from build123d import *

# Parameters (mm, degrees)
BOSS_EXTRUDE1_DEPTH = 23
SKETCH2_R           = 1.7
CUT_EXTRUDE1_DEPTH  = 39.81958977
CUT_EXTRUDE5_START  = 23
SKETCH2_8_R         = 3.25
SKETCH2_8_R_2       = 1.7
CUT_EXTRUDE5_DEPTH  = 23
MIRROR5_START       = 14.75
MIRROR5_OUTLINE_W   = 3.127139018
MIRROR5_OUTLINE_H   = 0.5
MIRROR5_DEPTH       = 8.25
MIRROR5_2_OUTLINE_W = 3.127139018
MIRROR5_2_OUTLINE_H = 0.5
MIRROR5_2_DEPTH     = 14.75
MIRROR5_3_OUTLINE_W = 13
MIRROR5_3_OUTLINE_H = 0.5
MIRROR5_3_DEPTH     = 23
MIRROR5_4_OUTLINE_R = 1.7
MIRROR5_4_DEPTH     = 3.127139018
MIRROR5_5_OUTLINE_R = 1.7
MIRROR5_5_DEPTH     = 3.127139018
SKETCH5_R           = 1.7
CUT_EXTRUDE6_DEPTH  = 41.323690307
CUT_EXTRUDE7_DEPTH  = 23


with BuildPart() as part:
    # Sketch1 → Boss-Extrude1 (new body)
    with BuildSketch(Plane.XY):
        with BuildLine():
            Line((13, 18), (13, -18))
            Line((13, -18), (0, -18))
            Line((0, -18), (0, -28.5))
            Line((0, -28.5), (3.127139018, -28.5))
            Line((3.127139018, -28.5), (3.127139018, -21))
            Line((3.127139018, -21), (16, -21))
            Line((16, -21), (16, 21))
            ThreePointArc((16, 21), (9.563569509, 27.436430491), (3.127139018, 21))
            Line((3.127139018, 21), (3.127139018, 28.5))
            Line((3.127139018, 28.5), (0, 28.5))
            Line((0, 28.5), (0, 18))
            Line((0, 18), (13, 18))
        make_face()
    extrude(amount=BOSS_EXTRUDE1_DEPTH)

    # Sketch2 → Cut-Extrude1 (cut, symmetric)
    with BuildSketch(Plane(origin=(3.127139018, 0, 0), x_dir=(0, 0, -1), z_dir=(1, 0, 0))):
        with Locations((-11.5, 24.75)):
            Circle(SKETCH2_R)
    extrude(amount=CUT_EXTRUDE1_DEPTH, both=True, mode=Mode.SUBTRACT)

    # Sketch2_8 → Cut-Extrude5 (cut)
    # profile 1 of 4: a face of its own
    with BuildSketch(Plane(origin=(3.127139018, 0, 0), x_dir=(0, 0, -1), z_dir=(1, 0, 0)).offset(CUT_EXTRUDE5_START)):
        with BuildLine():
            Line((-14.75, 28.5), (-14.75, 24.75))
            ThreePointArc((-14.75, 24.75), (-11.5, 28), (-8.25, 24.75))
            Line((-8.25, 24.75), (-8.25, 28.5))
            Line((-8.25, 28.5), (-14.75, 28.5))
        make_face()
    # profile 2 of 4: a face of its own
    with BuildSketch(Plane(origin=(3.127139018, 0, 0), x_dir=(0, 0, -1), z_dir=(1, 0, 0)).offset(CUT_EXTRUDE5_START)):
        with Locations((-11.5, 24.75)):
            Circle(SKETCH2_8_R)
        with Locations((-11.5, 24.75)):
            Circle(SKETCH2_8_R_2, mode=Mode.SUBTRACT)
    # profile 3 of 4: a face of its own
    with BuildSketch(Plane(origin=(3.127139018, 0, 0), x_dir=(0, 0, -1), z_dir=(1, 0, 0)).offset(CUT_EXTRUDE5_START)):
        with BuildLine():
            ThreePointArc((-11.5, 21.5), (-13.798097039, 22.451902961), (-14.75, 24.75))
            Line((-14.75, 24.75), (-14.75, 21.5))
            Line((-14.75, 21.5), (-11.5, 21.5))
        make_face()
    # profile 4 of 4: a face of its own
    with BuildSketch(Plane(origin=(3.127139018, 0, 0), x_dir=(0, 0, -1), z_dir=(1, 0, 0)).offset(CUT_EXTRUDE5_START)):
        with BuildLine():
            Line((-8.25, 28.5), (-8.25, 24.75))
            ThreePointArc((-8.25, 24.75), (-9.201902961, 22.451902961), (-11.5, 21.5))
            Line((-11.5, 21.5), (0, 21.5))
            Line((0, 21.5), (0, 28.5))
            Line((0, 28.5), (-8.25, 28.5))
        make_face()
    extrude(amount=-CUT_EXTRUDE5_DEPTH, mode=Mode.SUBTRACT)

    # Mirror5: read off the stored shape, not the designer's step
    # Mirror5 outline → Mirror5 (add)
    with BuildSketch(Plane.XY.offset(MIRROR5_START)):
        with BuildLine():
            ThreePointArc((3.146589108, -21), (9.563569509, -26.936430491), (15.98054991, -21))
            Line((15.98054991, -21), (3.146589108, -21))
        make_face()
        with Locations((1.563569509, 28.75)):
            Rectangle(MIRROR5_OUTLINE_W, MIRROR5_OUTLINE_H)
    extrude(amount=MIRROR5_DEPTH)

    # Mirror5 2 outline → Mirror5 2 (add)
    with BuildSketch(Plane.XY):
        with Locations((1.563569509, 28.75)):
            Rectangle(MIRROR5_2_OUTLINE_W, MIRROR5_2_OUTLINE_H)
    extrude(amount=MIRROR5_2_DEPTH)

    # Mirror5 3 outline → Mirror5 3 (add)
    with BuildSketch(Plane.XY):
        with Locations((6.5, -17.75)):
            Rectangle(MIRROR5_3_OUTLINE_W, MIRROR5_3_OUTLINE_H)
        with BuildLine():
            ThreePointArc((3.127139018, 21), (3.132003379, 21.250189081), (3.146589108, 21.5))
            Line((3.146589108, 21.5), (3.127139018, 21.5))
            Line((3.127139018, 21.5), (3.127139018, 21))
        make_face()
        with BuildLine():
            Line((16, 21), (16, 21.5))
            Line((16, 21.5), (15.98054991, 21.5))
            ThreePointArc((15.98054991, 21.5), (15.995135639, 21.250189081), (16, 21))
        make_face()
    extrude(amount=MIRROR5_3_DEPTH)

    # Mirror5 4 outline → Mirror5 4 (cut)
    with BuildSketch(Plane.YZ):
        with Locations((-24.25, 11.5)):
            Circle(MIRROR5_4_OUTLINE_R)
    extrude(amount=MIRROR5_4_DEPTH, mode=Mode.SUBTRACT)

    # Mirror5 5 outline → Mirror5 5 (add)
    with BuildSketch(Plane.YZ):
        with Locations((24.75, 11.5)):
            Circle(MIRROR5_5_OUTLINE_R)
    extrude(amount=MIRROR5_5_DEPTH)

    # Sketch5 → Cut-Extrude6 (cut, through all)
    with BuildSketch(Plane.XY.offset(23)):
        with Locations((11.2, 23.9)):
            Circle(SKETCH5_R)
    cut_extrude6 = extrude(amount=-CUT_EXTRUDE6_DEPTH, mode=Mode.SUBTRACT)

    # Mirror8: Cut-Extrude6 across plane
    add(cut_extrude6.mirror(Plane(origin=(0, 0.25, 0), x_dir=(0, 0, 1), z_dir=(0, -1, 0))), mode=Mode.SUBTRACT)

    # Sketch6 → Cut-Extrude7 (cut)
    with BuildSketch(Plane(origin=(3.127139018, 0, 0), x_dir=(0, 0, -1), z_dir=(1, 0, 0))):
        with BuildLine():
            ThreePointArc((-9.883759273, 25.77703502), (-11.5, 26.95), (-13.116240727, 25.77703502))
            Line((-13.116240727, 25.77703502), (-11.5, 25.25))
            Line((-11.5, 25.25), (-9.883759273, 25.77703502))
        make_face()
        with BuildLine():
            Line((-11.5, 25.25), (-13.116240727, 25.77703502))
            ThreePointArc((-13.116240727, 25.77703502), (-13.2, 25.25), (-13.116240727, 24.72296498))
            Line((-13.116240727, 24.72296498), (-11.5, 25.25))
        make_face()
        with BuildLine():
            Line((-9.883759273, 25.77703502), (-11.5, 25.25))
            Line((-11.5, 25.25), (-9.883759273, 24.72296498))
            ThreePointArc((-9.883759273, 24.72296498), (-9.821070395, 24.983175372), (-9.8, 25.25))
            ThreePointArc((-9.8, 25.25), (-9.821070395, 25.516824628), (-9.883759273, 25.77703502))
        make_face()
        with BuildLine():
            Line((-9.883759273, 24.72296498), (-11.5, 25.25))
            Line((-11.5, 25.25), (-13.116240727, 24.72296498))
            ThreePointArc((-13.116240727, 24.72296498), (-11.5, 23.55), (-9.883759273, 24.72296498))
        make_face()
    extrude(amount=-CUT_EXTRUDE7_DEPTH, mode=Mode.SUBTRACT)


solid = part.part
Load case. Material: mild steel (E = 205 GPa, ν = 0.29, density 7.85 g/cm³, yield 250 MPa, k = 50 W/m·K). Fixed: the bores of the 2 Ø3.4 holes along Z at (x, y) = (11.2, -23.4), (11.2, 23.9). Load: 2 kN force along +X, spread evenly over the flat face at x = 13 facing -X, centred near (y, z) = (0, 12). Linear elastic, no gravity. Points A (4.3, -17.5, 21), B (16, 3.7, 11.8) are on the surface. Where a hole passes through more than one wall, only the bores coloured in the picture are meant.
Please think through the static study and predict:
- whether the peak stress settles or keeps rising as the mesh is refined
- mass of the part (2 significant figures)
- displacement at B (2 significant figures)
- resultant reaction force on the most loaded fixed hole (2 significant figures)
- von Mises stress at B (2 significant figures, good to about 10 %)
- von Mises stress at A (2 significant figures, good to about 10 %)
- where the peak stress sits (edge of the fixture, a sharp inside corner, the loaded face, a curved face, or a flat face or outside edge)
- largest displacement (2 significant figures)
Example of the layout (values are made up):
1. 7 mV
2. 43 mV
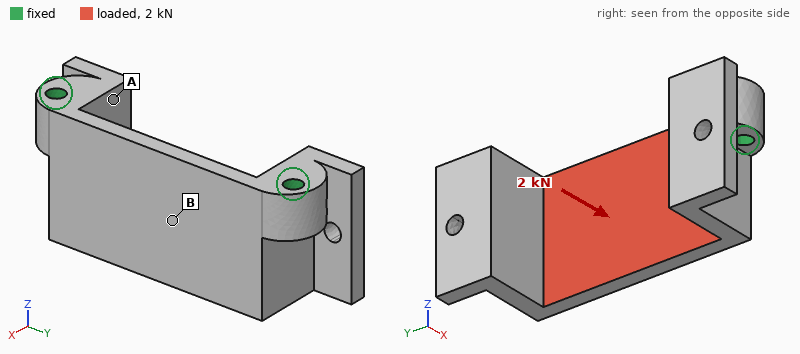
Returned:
1. keeps rising
2. 54 g
3. 42 µm
4. 1.3 kN
5. 110 MPa
6. 16 MPa
7. a sharp inside corner
8. 57 µm
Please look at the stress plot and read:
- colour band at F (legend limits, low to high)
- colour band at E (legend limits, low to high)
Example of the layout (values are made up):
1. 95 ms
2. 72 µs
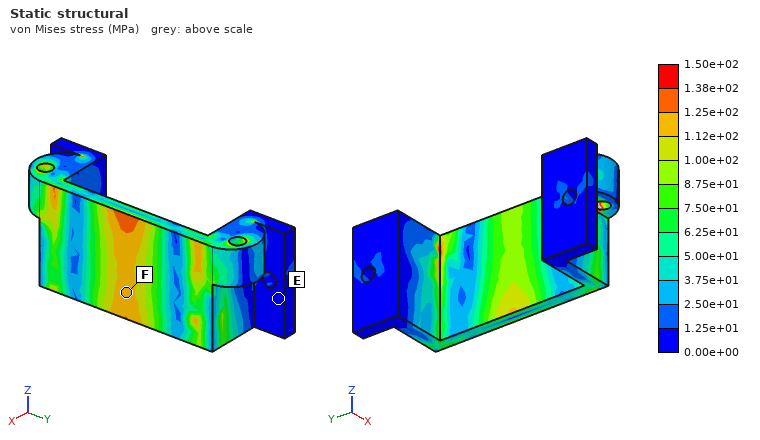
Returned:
1. 1.12e+02 to 1.25e+02 MPa
2. 0.00e+00 to 1.25e+01 MPa
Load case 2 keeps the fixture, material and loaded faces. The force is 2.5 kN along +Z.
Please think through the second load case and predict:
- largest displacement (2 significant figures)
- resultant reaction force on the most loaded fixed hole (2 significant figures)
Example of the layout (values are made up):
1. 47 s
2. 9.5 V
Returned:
1. 12 µm
2. 1.3 kN
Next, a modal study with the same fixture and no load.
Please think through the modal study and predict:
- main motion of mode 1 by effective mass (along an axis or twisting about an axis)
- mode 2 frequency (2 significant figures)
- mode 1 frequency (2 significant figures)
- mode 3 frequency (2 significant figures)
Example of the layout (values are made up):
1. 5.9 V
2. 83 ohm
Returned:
1. along X
2. 11 kHz
3. 7900 Hz
4. 11 kHz
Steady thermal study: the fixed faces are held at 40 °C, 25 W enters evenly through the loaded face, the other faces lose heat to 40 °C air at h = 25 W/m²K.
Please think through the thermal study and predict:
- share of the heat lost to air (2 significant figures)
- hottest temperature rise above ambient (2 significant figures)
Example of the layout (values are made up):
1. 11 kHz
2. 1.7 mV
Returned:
1. 8.6 %
2. 58 K
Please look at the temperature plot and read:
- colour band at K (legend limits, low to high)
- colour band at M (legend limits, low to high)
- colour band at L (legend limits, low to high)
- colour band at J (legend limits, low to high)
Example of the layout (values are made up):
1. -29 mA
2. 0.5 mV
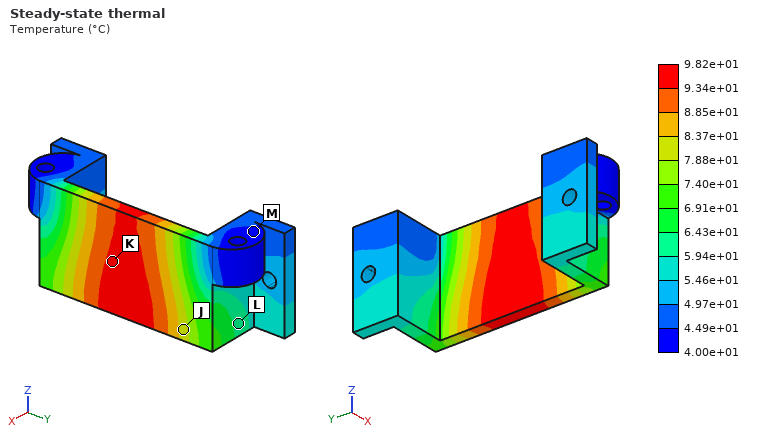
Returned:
1. 9.34e+01 to 9.82e+01 °C
2. 4.00e+01 to 4.49e+01 °C
3. 5.94e+01 to 6.43e+01 °C
4. 7.88e+01 to 8.37e+01 °C
